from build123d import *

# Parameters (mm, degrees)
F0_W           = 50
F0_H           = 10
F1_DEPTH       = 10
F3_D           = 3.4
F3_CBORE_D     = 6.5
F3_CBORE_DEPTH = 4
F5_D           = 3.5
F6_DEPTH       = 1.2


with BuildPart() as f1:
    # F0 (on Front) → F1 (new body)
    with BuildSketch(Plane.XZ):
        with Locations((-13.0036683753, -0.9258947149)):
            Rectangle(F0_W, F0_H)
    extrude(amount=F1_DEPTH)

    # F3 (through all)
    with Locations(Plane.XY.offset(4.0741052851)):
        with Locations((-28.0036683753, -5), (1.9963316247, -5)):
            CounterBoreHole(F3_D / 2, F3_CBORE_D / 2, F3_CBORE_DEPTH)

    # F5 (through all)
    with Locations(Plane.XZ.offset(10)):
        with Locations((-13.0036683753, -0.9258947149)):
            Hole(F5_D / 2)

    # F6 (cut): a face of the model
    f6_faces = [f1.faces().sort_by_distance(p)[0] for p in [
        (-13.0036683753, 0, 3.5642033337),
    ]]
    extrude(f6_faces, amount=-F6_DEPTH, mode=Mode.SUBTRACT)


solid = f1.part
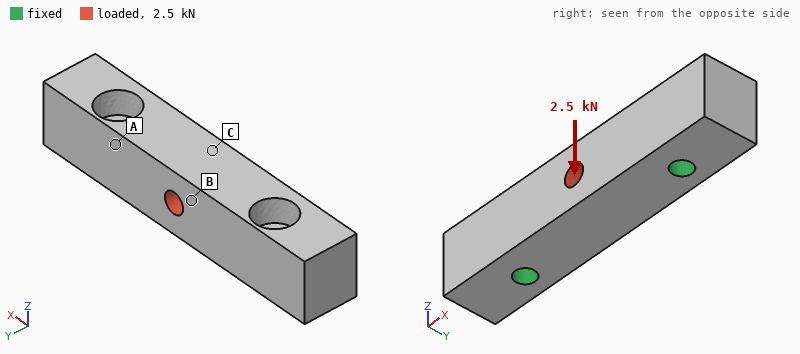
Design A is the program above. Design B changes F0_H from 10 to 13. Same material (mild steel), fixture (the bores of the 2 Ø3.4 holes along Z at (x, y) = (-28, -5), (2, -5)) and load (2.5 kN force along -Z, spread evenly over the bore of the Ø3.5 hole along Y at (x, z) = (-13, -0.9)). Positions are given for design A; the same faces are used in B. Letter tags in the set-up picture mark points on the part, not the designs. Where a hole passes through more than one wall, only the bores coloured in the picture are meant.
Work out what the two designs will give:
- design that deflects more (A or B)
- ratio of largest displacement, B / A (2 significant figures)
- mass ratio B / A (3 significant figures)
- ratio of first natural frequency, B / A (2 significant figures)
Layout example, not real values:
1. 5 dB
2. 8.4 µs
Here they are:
1. A
2. 0.63
3. 1.30
4. 0.95
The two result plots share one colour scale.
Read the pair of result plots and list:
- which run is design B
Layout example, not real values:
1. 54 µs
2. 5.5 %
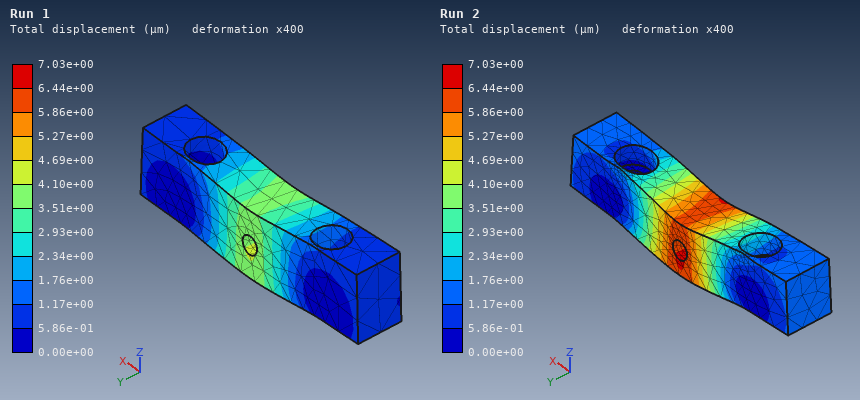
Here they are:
1. Run 1
